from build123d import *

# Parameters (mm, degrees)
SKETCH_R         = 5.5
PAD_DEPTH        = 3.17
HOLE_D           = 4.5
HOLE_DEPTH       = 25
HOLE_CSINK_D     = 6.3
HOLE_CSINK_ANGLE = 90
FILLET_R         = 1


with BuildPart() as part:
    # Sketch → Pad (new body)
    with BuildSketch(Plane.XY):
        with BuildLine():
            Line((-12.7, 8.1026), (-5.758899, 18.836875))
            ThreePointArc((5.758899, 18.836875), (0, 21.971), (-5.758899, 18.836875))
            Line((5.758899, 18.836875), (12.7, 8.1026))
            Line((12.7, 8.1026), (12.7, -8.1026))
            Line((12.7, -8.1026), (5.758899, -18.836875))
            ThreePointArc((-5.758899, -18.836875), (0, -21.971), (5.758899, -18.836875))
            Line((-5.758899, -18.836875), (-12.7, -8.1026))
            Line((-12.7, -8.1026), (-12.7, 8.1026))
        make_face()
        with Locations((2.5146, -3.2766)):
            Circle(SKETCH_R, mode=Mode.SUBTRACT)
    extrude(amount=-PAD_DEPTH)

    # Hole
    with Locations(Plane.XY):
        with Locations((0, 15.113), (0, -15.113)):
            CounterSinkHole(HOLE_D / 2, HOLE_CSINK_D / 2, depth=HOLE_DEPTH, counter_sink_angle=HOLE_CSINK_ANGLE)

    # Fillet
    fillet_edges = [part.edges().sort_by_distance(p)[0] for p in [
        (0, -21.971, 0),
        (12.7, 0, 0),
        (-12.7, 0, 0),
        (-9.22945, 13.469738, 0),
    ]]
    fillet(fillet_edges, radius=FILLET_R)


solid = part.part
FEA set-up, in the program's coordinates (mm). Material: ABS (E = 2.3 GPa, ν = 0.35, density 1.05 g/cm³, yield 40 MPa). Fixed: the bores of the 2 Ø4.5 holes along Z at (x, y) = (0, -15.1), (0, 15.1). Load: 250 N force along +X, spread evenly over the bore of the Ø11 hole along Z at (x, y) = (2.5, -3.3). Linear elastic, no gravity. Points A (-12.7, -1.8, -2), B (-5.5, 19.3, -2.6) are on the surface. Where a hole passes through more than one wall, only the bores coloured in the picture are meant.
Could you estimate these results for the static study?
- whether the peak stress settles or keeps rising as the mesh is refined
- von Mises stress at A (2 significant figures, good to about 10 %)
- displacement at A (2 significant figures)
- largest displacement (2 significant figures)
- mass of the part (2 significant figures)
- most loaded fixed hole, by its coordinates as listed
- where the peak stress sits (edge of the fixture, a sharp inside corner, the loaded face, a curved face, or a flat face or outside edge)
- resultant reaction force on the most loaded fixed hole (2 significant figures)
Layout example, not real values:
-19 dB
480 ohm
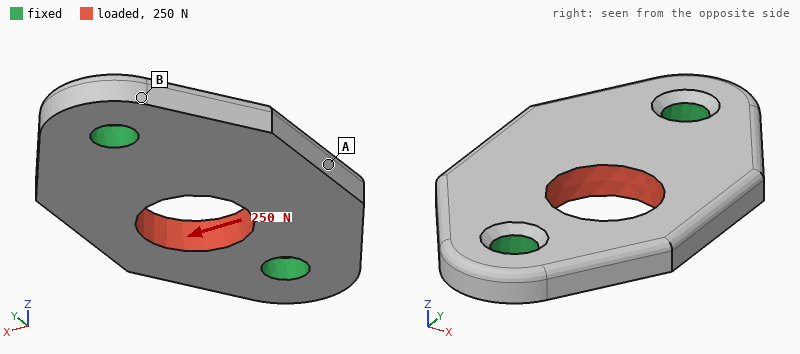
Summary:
keeps rising
4.5 MPa
32 µm
51 µm
2.4 g
(0, -15.1)
edge of the fixture
150 N
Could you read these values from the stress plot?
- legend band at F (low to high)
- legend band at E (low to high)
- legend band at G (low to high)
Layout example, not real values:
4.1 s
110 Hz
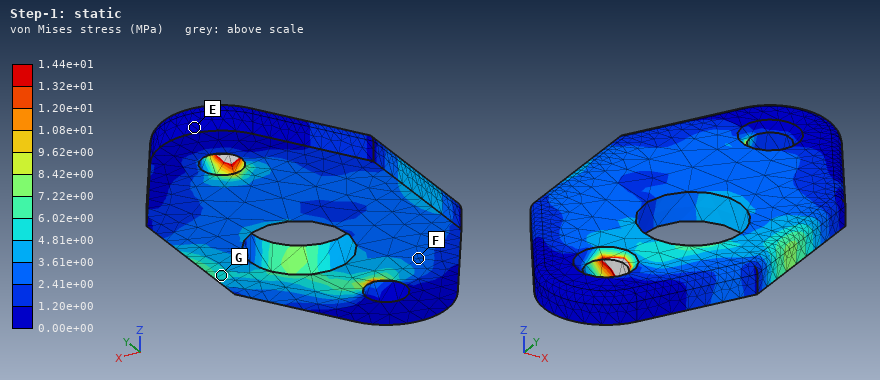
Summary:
2.41e+00 to 3.61e+00 MPa
0.00e+00 to 1.20e+00 MPa
4.81e+00 to 6.02e+00 MPa
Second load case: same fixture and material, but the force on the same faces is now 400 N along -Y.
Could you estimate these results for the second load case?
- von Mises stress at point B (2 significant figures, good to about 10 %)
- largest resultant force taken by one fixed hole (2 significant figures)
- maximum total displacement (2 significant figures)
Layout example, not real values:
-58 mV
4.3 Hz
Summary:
1.9 MPa
210 N
50 µm
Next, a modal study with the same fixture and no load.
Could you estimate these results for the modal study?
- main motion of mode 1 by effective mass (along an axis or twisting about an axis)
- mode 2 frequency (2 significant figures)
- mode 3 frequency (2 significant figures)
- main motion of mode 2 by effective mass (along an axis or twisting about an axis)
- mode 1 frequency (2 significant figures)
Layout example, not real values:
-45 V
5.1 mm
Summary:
twisting about Y
3700 Hz
7700 Hz
along Z
3300 Hz
